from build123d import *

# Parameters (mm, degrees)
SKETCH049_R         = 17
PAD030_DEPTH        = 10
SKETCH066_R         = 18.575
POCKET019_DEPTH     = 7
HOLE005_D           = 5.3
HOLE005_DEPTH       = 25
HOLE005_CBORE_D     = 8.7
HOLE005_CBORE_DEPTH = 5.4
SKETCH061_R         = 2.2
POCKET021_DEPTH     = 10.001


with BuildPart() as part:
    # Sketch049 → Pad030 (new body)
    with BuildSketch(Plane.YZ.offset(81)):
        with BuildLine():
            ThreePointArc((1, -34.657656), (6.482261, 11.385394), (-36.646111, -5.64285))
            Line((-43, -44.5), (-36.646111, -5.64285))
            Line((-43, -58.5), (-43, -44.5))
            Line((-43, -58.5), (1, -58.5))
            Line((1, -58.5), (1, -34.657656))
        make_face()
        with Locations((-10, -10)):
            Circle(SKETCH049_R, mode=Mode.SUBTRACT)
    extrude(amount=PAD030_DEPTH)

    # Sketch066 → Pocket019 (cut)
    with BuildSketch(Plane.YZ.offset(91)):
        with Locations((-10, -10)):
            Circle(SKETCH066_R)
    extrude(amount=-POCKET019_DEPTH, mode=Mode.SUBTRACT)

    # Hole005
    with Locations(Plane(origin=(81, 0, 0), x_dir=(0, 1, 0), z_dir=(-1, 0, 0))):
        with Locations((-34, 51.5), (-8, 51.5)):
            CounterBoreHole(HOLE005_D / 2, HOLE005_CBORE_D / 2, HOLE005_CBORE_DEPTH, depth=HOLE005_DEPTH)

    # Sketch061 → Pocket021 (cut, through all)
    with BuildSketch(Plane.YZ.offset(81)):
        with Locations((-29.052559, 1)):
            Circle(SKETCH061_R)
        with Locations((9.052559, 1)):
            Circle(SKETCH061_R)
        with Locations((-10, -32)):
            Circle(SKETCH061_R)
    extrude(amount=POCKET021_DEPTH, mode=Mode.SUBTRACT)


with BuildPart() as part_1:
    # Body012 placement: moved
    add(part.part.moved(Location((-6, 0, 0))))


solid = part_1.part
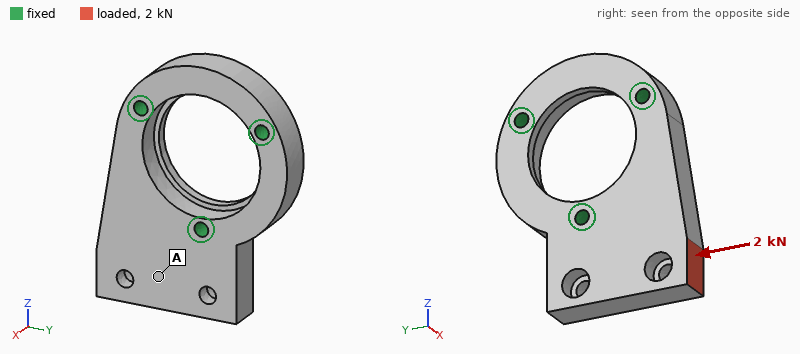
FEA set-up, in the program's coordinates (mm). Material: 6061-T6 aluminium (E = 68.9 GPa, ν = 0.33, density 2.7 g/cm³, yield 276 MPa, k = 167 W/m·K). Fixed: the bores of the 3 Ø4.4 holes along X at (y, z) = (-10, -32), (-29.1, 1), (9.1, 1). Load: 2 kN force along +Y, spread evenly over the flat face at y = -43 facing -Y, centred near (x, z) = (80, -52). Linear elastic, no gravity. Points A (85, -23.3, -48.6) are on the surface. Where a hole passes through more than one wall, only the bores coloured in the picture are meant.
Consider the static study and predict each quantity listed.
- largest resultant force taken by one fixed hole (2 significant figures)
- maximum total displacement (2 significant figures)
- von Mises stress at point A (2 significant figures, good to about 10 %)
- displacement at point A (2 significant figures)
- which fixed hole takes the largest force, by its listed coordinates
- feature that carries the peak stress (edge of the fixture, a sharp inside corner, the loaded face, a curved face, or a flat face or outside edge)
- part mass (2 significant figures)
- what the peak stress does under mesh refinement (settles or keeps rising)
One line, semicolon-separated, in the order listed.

2.3 kN; 24 µm; 9.7 MPa; 9.8 µm; (-10, -32); edge of the fixture; 62 g; keeps rising
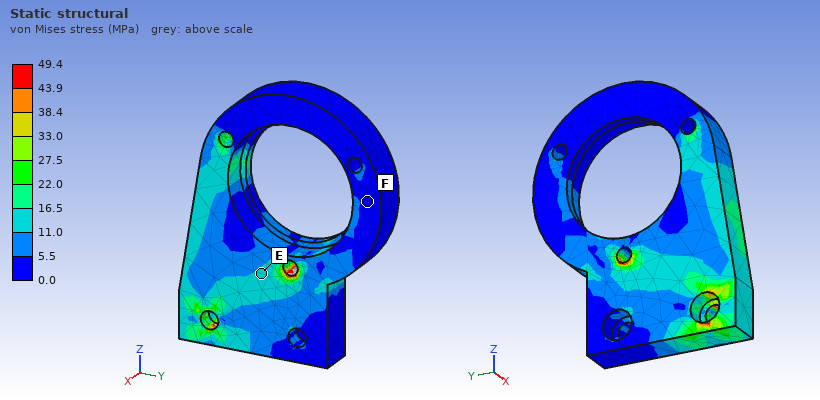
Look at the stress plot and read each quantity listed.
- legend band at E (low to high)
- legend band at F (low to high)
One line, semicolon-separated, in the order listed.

11.0 to 16.5 MPa; 0.0 to 5.5 MPa
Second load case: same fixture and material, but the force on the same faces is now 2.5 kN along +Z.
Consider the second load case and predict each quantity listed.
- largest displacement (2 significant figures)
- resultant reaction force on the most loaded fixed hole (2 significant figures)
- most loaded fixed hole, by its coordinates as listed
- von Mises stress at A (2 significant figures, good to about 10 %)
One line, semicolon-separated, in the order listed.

40 µm; 2.7 kN; (-29.1, 1); 5.4 MPa
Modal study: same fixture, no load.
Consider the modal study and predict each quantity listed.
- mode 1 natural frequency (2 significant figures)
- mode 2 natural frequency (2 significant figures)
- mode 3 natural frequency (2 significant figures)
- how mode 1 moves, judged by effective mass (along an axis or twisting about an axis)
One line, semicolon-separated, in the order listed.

5400 Hz; 11 kHz; 13 kHz; along X
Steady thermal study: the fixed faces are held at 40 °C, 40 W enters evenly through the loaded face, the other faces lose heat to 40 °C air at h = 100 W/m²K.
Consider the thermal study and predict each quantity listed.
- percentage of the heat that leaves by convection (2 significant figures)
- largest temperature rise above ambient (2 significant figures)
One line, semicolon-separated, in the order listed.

15 %; 42 K
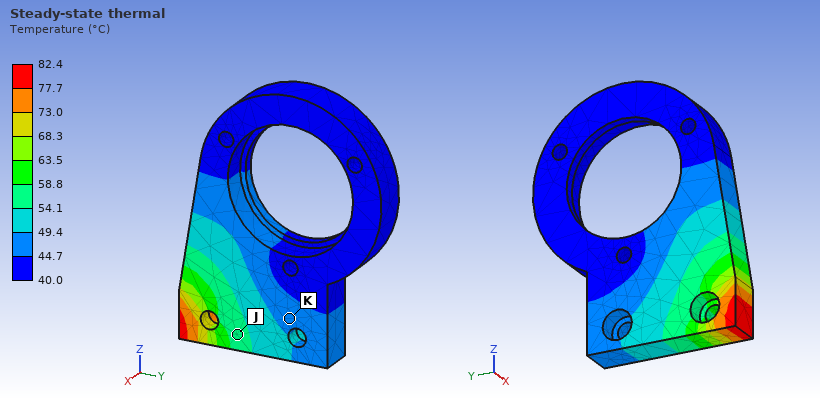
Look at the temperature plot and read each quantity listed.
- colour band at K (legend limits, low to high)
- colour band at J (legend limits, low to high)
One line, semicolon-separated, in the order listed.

44.7 to 49.4 °C; 54.1 to 58.8 °C
